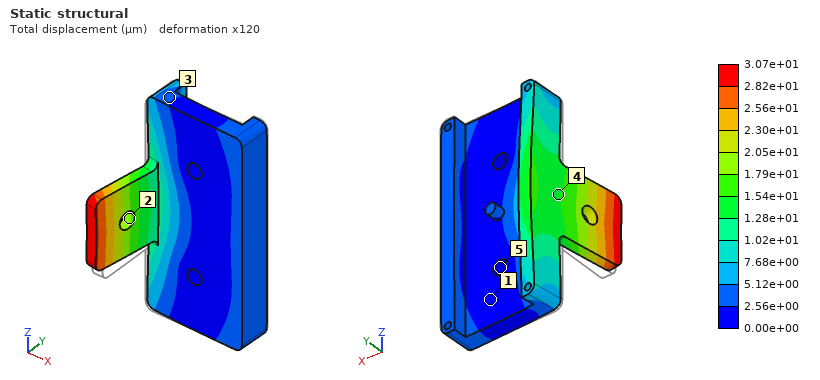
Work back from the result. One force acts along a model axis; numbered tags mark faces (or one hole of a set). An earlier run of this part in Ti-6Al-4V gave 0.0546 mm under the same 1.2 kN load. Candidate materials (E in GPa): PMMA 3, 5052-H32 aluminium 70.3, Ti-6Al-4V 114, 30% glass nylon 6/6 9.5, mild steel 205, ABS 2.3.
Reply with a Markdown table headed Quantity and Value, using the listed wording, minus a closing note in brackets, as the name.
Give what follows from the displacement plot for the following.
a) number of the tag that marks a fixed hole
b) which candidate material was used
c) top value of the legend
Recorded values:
| Quantity | Value |
|---|---|
| number of the tag that marks a fixed hole | 5 |
| which candidate material was used | mild steel |
| top value of the legend | 3.07e+01 µm |
